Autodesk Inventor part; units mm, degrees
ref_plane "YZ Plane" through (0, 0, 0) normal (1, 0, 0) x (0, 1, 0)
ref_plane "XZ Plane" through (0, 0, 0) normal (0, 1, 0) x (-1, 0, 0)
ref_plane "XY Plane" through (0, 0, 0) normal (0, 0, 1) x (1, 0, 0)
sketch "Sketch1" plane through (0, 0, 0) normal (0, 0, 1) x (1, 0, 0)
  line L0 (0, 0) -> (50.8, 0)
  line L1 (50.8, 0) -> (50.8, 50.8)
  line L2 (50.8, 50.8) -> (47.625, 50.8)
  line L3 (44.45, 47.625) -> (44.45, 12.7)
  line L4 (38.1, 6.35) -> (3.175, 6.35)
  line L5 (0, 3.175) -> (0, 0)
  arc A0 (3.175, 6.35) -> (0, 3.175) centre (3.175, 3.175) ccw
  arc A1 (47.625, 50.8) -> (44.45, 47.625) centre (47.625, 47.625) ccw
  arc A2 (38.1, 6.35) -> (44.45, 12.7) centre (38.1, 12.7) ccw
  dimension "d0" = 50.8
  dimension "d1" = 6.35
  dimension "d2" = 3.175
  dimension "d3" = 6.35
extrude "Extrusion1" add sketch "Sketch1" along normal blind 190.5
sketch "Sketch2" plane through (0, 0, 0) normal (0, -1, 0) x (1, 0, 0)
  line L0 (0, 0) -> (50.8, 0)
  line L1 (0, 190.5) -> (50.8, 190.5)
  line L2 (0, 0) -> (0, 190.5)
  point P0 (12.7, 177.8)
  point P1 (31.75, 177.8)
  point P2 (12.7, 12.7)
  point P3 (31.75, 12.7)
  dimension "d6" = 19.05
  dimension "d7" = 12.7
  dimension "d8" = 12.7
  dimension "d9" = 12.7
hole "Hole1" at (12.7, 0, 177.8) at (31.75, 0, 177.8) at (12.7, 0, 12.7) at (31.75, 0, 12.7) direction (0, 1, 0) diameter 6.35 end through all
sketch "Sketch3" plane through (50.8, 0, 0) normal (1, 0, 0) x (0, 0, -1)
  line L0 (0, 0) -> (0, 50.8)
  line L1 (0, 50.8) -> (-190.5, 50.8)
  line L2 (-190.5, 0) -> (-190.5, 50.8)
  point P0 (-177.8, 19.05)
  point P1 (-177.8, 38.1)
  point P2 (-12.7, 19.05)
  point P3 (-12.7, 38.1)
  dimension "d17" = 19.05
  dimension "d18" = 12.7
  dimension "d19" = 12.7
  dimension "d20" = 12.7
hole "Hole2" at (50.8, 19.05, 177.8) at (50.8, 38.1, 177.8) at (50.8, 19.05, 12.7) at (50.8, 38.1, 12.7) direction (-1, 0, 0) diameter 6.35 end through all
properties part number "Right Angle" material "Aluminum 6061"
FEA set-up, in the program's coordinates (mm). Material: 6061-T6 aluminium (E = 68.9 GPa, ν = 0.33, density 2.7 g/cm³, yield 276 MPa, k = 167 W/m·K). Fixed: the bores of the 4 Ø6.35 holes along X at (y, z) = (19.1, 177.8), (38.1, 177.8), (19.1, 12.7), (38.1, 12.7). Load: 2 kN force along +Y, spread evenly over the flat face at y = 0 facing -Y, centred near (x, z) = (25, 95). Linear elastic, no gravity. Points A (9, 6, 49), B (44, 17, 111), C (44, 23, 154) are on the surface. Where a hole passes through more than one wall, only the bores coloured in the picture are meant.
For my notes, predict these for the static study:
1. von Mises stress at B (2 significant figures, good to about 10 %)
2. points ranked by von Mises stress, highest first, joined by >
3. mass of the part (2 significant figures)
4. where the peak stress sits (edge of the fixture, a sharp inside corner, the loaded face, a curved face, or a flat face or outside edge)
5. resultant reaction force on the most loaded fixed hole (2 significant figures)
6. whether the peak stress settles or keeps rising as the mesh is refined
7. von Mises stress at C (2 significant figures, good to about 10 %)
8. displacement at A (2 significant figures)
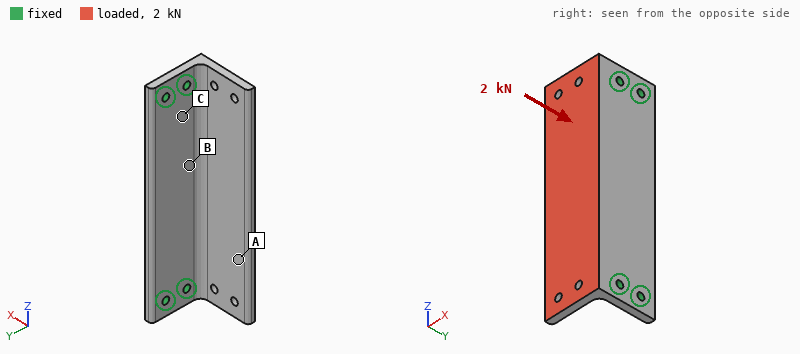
16 MPa
C > B > A
310 g
edge of the fixture
1.1 kN
keeps rising
30 MPa
0.20 mm
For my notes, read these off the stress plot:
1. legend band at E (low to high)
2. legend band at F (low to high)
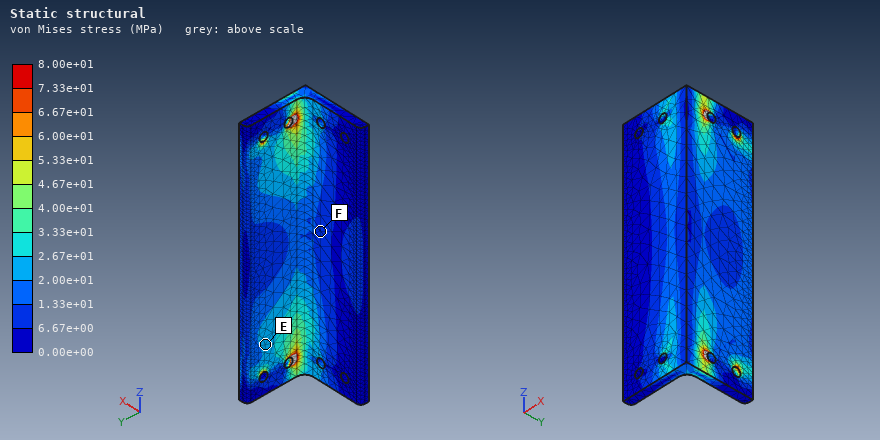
2.00e+01 to 2.67e+01 MPa
6.67e+00 to 1.33e+01 MPa
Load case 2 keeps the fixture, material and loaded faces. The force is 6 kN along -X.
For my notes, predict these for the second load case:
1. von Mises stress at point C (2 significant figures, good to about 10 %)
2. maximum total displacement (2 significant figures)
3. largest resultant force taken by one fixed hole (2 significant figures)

47 MPa
0.39 mm
4.6 kN
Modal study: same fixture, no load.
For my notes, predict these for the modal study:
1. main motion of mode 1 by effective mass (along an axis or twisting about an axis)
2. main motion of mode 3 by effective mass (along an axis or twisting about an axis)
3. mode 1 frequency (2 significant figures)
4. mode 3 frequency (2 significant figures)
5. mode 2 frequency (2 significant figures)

along Y
along X
1200 Hz
2300 Hz
2100 Hz
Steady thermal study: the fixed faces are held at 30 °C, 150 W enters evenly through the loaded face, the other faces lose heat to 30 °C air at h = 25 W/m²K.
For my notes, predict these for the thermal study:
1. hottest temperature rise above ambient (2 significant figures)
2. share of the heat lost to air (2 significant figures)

49 K
13 %
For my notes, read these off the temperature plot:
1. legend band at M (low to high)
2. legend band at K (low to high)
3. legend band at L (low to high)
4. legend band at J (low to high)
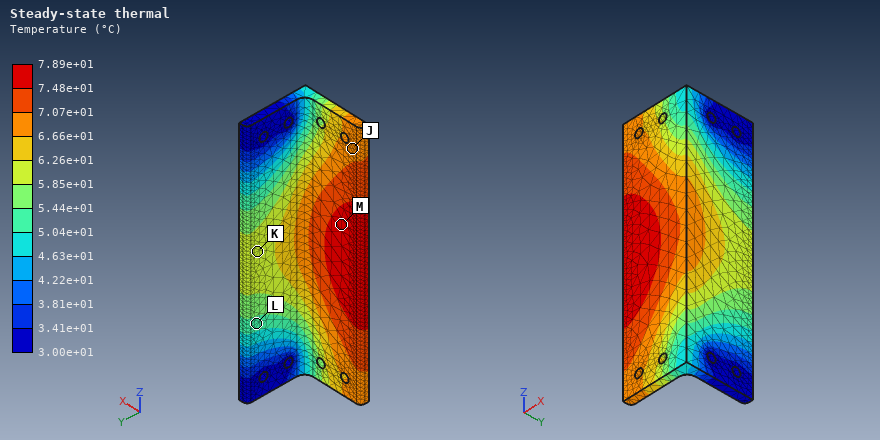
7.48e+01 to 7.89e+01 °C
5.85e+01 to 6.26e+01 °C
5.04e+01 to 5.44e+01 °C
6.66e+01 to 7.07e+01 °C
